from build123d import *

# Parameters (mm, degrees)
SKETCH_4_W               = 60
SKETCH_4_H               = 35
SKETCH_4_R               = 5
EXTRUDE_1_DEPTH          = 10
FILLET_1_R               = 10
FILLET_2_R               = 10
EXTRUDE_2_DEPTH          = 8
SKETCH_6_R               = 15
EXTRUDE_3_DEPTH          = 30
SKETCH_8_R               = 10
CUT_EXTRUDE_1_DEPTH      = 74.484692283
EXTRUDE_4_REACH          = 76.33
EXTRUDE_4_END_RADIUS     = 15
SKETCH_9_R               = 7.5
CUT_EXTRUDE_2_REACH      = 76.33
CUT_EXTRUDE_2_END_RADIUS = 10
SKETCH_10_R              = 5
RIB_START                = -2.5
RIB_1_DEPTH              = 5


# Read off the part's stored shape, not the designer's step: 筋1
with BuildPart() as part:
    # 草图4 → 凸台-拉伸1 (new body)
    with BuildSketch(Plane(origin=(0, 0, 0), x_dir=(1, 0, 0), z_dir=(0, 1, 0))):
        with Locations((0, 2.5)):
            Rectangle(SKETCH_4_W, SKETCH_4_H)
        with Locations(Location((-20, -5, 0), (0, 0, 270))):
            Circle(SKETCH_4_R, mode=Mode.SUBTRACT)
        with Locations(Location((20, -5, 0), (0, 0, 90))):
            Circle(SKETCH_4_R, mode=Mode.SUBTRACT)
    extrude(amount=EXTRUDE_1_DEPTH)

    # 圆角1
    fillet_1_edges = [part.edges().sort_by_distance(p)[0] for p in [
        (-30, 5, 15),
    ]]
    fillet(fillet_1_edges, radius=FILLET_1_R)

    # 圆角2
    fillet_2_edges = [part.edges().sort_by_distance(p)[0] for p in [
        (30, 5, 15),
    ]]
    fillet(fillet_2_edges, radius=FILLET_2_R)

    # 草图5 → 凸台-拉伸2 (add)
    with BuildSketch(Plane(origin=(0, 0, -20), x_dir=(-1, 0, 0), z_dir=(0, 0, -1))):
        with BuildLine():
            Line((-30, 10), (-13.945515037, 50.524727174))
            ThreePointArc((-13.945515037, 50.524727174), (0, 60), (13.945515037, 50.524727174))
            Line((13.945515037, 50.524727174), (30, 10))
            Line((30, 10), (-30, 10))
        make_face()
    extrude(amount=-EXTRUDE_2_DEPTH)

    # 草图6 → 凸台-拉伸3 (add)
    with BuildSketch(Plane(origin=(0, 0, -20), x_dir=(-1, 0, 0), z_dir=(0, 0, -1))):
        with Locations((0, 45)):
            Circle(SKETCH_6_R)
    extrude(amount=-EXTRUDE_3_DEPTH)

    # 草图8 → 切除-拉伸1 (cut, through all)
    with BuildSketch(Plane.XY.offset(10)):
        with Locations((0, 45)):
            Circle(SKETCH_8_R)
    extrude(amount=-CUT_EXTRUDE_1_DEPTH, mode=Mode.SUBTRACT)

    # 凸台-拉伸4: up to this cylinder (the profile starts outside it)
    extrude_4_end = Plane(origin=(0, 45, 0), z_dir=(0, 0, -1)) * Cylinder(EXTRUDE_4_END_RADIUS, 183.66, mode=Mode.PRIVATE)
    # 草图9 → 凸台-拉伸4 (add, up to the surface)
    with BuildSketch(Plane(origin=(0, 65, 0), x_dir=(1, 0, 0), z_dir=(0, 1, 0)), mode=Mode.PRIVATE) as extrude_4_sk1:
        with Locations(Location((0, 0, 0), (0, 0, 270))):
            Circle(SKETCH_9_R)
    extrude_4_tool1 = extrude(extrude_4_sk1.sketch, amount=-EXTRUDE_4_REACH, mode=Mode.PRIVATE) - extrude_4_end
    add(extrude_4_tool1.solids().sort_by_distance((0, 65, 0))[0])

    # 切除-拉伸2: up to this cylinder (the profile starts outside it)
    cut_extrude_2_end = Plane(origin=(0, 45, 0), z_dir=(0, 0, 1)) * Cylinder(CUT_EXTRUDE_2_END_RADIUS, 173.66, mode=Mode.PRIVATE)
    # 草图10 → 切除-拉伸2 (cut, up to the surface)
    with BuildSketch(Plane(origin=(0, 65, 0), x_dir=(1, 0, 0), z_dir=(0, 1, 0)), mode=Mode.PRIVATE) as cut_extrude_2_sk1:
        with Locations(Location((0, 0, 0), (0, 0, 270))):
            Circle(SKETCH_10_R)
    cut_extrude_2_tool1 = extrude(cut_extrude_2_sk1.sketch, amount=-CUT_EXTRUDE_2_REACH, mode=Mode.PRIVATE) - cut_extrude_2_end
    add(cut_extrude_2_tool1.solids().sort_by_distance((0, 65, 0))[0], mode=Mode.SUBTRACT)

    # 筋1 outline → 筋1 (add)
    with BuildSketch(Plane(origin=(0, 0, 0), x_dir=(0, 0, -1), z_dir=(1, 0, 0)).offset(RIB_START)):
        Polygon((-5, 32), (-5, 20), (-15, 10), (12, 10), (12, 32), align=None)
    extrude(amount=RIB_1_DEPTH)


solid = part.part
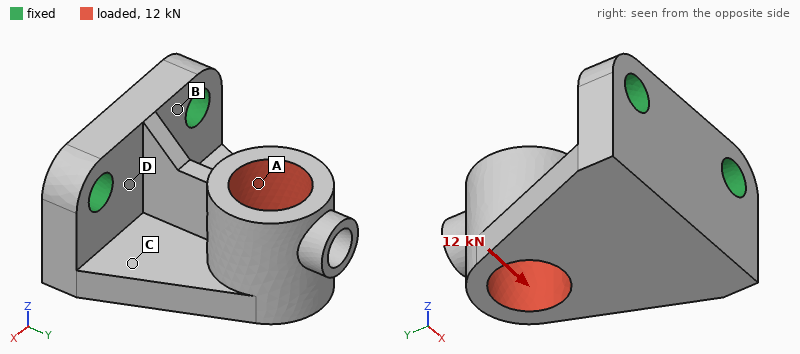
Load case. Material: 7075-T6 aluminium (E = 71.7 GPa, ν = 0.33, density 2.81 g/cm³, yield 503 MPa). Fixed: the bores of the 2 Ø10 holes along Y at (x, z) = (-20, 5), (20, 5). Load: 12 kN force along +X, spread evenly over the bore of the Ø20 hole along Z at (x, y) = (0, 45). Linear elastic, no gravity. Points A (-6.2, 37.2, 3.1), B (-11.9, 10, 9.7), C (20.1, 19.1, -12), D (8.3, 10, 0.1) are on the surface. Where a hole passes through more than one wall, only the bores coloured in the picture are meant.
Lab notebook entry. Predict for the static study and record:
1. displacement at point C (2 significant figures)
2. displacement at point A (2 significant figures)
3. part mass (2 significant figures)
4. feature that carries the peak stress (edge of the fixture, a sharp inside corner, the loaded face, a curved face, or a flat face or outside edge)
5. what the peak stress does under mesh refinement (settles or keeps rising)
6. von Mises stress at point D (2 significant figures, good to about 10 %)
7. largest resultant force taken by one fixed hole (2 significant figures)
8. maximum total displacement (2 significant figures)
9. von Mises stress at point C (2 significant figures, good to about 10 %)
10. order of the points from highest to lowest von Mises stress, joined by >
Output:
0.17 mm
0.45 mm
120 g
edge of the fixture
keeps rising
130 MPa
13 kN
0.73 mm
170 MPa
C > D > A > B
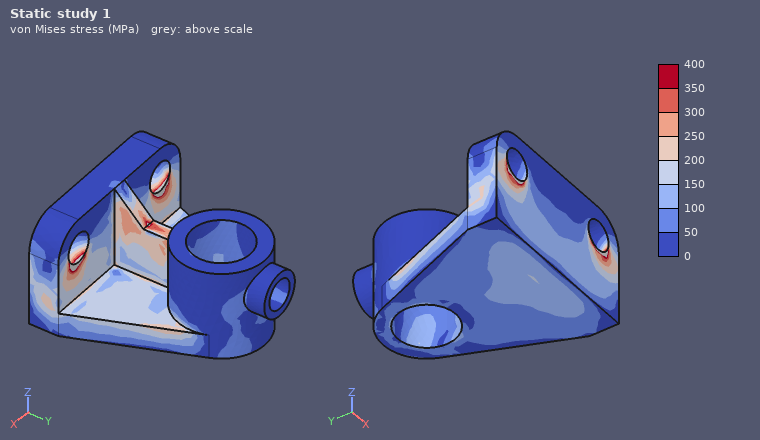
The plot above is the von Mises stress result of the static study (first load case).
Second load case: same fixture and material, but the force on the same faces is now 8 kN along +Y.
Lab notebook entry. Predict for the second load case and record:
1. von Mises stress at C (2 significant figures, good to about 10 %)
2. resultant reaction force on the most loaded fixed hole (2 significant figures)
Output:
37 MPa
4.0 kN
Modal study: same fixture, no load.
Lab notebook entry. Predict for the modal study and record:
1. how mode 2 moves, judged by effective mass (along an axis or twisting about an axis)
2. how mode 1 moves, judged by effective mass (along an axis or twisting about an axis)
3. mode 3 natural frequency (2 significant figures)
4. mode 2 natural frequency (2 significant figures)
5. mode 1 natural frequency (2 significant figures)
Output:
along X
along Z
7700 Hz
3800 Hz
3000 Hz
